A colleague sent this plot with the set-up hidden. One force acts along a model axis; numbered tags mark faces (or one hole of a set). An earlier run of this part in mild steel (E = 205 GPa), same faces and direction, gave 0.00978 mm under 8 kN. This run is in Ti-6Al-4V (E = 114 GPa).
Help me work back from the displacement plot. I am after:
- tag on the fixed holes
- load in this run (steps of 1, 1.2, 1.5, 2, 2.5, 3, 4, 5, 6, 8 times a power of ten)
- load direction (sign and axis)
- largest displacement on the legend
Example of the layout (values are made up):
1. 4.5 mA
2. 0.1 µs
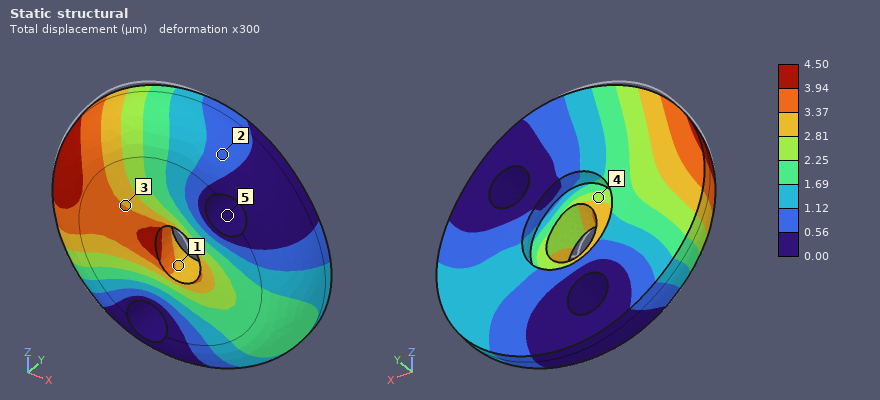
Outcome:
1. 5
2. 2 kN
3. +X
4. 4.50 µm
